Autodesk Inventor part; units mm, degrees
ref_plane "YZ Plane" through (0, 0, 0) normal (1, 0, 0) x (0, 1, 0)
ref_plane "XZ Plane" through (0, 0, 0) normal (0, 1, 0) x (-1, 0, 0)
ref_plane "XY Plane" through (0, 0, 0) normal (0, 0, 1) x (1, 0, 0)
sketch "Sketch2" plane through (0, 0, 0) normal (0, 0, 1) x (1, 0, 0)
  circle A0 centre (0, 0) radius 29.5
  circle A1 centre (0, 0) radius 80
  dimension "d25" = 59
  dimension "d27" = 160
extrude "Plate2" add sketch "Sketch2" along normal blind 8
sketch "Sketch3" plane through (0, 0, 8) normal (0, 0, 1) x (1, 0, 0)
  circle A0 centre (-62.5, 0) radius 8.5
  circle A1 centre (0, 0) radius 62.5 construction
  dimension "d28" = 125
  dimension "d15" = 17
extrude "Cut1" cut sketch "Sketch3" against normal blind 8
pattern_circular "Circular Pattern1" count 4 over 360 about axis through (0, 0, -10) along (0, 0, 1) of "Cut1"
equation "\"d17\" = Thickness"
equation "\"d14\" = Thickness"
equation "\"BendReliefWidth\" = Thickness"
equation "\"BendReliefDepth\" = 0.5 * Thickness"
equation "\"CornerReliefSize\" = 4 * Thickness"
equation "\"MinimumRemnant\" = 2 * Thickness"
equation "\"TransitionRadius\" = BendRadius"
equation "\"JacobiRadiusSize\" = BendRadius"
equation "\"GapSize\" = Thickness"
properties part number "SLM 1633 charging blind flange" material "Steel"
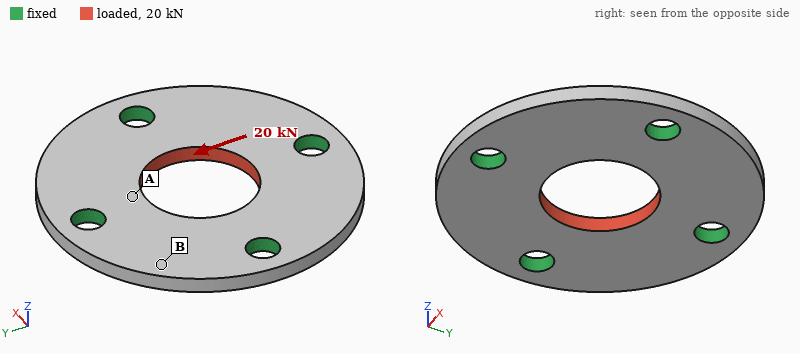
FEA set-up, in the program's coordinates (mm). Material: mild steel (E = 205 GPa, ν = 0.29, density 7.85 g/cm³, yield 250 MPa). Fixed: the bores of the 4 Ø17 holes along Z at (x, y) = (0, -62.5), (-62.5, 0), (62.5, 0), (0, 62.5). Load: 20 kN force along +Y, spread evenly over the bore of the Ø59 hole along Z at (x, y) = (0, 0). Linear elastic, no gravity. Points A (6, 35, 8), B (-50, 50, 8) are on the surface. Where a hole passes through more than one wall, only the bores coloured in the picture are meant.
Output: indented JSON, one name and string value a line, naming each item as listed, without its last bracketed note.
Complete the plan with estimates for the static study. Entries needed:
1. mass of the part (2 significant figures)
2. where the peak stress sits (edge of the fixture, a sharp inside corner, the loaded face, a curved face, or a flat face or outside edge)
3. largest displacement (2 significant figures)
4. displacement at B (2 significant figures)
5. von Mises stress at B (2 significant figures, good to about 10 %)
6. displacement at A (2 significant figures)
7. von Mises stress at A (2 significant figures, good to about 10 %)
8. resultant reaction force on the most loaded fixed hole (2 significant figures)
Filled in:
{
  "mass of the part": "1.0 kg",
  "where the peak stress sits": "edge of the fixture",
  "largest displacement": "4.0 µm",
  "displacement at B": "2.1 µm",
  "von Mises stress at B": "5.7 MPa",
  "displacement at A": "2.1 µm",
  "von Mises stress at A": "19 MPa",
  "resultant reaction force on the most loaded fixed hole": "5.8 kN"
}
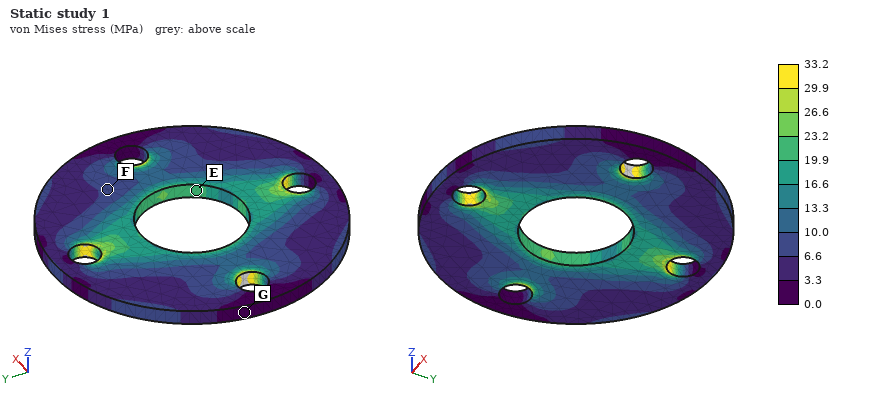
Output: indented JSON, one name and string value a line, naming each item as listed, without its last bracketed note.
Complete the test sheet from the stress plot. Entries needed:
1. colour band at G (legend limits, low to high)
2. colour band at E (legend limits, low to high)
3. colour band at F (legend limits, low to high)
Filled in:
{
  "colour band at G": "0.0 to 3.3 MPa",
  "colour band at E": "19.9 to 23.2 MPa",
  "colour band at F": "6.6 to 10.0 MPa"
}
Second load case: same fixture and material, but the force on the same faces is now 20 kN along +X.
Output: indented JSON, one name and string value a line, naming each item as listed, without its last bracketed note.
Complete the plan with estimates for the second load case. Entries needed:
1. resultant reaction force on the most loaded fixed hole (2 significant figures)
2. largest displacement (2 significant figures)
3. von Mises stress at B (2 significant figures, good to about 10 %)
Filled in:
{
  "resultant reaction force on the most loaded fixed hole": "5.8 kN",
  "largest displacement": "4.0 µm",
  "von Mises stress at B": "5.7 MPa"
}
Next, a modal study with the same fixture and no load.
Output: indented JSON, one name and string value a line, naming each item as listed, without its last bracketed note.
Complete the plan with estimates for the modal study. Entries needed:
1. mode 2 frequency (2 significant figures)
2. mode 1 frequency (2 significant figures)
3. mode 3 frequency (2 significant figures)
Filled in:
{
  "mode 2 frequency": "4800 Hz",
  "mode 1 frequency": "4700 Hz",
  "mode 3 frequency": "4800 Hz"
}
